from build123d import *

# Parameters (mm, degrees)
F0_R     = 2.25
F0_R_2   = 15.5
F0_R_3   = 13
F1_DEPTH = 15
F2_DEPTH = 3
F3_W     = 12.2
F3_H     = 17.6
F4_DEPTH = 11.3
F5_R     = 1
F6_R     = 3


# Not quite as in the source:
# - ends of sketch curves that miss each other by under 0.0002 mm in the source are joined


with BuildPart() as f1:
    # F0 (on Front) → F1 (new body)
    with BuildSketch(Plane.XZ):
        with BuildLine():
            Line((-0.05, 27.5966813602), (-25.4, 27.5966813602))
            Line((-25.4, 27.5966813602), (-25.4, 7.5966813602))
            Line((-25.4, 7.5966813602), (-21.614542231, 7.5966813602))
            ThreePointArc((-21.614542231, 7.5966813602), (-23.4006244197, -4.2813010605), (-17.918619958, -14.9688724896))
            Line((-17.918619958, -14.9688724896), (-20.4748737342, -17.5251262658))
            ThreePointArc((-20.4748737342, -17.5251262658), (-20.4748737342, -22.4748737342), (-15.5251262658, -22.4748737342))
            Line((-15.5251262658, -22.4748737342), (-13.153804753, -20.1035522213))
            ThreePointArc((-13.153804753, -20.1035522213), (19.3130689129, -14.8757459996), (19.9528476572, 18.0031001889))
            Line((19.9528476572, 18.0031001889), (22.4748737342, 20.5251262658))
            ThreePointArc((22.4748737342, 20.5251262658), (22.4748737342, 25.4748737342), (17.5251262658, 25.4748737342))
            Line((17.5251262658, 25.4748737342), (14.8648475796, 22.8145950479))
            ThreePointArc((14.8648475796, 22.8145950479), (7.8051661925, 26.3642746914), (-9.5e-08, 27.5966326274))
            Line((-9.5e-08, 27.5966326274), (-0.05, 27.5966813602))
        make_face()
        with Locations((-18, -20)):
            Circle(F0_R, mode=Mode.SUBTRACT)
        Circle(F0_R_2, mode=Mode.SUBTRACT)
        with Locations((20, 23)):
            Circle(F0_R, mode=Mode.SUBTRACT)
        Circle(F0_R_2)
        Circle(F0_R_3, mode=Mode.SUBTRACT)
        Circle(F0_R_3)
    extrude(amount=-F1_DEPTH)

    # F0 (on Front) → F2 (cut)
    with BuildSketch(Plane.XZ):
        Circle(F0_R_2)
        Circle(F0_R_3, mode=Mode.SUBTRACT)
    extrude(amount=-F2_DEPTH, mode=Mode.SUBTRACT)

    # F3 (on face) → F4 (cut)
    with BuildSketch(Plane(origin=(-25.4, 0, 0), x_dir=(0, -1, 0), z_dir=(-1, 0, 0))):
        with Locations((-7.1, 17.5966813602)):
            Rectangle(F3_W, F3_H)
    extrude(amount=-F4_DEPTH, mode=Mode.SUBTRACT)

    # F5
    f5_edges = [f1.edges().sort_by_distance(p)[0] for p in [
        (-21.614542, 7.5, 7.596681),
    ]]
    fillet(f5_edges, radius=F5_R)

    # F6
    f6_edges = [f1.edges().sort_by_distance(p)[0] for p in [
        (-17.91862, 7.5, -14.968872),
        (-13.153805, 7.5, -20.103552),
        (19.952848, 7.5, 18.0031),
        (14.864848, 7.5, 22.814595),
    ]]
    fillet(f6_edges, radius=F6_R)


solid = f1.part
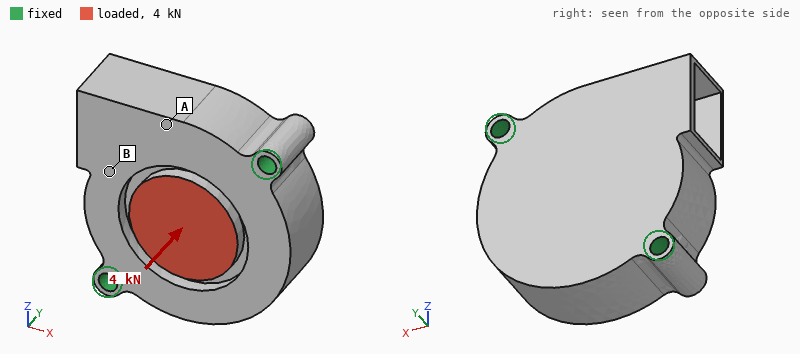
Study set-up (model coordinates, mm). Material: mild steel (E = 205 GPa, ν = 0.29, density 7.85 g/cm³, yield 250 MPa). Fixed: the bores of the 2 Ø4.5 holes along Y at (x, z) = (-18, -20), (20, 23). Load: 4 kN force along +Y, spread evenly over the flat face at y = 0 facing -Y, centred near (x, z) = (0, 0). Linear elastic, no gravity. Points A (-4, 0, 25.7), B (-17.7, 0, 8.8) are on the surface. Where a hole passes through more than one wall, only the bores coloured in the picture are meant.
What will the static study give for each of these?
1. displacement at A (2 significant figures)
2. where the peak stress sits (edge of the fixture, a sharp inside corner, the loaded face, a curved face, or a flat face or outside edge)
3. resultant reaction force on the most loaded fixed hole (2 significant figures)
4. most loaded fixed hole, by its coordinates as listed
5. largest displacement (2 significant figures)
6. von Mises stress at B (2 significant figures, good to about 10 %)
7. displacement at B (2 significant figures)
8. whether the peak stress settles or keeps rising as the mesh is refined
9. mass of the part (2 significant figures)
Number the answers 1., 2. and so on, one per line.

1. 3.6 µm
2. edge of the fixture
3. 2.2 kN
4. (-18, -20)
5. 5.4 µm
6. 18 MPa
7. 4.4 µm
8. keeps rising
9. 240 g
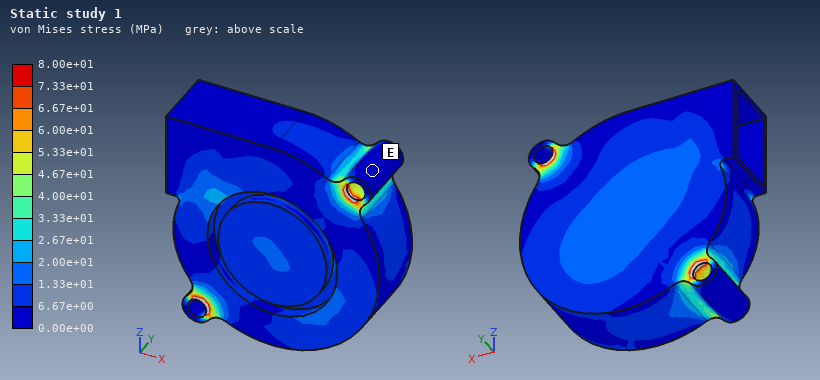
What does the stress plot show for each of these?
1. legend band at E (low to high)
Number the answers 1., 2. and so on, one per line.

1. 0.00e+00 to 6.67e+00 MPa
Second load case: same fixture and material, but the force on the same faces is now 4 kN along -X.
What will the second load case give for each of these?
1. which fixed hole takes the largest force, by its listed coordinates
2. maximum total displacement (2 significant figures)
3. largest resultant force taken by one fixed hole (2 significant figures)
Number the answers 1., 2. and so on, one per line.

1. (-18, -20)
2. 10 µm
3. 2.2 kN
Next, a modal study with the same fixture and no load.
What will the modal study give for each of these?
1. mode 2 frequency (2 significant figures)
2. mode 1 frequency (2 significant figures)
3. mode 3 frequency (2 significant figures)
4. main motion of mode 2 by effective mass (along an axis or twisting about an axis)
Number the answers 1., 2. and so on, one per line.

1. 10 kHz
2. 6900 Hz
3. 15 kHz
4. along Y
